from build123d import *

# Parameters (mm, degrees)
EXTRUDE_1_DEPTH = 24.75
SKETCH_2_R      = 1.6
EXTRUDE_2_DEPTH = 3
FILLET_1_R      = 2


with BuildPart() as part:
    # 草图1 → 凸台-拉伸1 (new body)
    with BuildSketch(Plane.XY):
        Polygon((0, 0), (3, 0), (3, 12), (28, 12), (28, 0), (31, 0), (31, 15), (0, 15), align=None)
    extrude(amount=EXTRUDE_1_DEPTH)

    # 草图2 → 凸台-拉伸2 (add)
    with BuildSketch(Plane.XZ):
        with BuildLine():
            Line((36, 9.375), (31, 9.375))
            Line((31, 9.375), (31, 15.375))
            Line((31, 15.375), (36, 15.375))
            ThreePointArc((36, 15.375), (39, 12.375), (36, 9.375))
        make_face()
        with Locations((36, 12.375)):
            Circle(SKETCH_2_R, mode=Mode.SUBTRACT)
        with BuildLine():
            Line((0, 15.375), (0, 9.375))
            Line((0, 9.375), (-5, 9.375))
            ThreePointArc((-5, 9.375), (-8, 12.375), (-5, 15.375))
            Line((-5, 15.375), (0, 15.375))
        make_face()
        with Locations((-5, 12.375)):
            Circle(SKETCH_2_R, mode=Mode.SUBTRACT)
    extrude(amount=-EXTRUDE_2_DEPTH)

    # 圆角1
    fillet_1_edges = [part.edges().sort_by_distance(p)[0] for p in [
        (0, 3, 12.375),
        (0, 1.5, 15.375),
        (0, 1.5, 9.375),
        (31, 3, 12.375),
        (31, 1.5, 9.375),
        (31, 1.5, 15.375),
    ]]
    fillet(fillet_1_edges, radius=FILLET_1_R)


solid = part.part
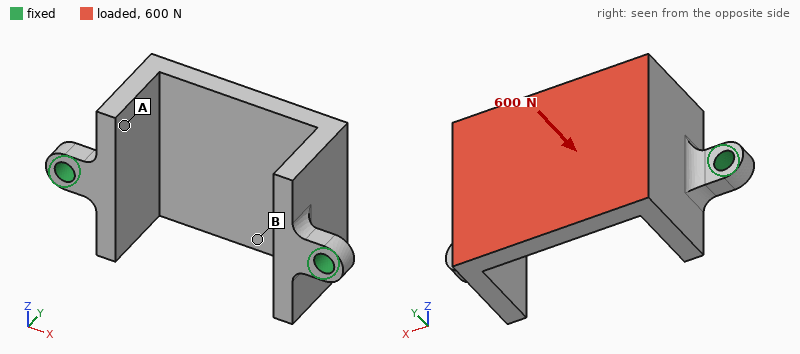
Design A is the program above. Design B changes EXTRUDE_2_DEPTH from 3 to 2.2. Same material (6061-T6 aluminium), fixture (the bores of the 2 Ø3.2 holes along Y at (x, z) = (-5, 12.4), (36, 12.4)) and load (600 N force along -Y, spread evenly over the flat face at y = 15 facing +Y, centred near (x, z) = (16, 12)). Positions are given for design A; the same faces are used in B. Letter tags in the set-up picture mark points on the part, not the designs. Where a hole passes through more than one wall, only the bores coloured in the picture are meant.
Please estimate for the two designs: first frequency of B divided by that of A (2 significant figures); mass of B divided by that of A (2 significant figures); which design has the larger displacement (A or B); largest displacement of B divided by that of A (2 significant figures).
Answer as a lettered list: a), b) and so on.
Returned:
a) 0.73
b) 0.99
c) B
d) 1.2
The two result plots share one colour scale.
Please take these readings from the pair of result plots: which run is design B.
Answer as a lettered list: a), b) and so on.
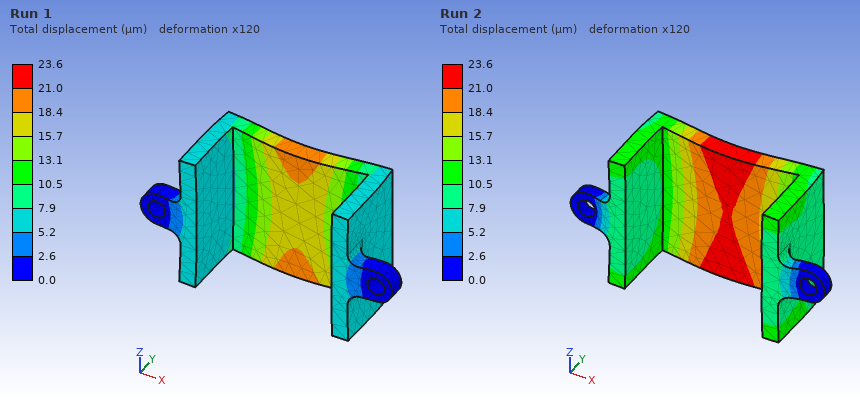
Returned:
a) Run 2
